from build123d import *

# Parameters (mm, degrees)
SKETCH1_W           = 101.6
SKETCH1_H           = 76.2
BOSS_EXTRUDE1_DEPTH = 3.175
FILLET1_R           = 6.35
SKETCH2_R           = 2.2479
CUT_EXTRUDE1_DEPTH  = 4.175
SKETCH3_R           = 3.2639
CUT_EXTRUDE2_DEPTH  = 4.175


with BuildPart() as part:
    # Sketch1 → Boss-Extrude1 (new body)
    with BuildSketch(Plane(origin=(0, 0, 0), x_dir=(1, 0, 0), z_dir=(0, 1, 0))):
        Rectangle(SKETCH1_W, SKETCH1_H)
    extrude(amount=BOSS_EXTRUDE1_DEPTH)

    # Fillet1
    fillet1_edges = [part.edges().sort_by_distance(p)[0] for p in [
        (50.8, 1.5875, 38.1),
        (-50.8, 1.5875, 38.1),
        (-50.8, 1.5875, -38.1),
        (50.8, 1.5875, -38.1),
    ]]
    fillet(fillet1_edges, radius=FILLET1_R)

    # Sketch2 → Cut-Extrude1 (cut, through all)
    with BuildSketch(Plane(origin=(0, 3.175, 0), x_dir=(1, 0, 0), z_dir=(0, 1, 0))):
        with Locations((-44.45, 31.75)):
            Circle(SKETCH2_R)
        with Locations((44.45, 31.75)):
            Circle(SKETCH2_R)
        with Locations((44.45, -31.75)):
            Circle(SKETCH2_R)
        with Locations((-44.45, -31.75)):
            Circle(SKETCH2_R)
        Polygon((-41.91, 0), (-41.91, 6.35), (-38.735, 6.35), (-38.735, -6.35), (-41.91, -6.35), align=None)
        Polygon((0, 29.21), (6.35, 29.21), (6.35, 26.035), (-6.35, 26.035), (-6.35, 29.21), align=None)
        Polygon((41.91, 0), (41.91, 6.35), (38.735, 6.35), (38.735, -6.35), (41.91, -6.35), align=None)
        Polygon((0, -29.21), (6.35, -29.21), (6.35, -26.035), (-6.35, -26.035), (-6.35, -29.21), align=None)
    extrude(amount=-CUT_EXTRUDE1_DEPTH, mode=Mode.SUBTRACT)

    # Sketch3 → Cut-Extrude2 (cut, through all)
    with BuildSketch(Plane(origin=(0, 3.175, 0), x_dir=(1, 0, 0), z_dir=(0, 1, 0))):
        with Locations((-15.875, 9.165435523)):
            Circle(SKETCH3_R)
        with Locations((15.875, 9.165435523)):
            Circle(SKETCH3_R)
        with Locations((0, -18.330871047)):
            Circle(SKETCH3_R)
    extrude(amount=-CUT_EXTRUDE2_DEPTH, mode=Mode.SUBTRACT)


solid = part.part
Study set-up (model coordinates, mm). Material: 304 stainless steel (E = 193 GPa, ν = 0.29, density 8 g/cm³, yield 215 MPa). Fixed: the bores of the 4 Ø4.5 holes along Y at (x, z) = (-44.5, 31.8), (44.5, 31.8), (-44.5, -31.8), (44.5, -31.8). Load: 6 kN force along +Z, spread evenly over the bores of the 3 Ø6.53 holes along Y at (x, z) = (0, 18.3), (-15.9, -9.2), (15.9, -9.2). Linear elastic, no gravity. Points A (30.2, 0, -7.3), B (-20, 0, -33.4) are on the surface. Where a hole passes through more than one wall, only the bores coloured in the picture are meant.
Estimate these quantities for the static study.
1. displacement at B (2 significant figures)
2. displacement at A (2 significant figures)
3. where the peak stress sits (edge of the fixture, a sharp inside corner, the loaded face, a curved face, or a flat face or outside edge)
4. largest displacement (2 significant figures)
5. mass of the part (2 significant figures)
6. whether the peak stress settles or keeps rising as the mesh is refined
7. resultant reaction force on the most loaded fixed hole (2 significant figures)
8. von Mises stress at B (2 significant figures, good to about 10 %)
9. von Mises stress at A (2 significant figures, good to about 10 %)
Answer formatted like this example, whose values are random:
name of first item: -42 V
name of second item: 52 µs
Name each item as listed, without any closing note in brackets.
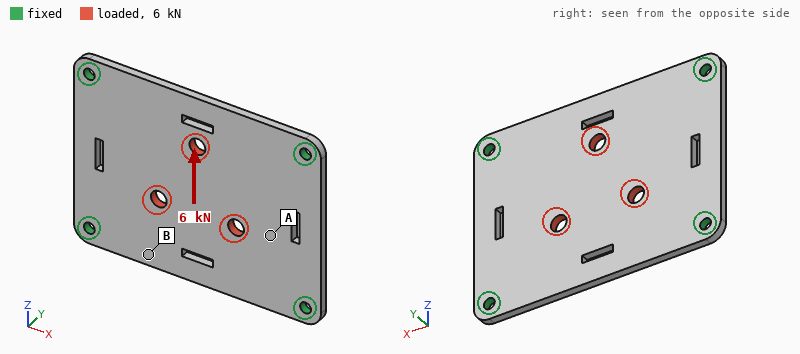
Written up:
displacement at B: 6.8 µm
displacement at A: 4.9 µm
where the peak stress sits: edge of the fixture
largest displacement: 11 µm
mass of the part: 190 g
whether the peak stress settles or keeps rising as the mesh is refined: keeps rising
resultant reaction force on the most loaded fixed hole: 1.8 kN
von Mises stress at B: 9.6 MPa
von Mises stress at A: 27 MPa
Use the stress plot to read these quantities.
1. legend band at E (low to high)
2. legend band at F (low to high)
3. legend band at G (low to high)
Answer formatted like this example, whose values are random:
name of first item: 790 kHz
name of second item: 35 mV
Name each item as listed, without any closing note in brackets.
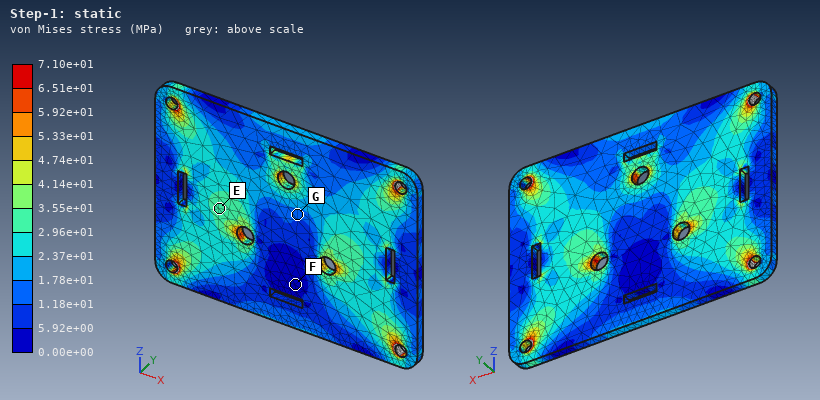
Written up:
legend band at E: 2.96e+01 to 3.55e+01 MPa
legend band at F: 0.00e+00 to 5.92e+00 MPa
legend band at G: 1.18e+01 to 1.78e+01 MPa
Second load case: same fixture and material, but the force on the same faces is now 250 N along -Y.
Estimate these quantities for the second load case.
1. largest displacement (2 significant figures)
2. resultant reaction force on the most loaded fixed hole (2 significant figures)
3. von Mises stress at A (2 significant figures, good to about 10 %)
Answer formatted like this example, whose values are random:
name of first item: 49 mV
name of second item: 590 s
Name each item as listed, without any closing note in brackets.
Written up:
largest displacement: 34 µm
resultant reaction force on the most loaded fixed hole: 63 N
von Mises stress at A: 9.2 MPa
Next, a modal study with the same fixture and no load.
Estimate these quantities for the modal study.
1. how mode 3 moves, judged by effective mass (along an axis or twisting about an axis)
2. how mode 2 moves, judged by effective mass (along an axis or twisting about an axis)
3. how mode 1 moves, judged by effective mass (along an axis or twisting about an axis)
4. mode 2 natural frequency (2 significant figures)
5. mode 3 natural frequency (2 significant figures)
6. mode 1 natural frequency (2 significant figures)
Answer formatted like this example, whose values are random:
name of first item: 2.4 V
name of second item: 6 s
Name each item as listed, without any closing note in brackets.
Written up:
how mode 3 moves, judged by effective mass: twisting about Z
how mode 2 moves, judged by effective mass: twisting about X
how mode 1 moves, judged by effective mass: along Y
mode 2 natural frequency: 2600 Hz
mode 3 natural frequency: 3700 Hz
mode 1 natural frequency: 1600 Hz
